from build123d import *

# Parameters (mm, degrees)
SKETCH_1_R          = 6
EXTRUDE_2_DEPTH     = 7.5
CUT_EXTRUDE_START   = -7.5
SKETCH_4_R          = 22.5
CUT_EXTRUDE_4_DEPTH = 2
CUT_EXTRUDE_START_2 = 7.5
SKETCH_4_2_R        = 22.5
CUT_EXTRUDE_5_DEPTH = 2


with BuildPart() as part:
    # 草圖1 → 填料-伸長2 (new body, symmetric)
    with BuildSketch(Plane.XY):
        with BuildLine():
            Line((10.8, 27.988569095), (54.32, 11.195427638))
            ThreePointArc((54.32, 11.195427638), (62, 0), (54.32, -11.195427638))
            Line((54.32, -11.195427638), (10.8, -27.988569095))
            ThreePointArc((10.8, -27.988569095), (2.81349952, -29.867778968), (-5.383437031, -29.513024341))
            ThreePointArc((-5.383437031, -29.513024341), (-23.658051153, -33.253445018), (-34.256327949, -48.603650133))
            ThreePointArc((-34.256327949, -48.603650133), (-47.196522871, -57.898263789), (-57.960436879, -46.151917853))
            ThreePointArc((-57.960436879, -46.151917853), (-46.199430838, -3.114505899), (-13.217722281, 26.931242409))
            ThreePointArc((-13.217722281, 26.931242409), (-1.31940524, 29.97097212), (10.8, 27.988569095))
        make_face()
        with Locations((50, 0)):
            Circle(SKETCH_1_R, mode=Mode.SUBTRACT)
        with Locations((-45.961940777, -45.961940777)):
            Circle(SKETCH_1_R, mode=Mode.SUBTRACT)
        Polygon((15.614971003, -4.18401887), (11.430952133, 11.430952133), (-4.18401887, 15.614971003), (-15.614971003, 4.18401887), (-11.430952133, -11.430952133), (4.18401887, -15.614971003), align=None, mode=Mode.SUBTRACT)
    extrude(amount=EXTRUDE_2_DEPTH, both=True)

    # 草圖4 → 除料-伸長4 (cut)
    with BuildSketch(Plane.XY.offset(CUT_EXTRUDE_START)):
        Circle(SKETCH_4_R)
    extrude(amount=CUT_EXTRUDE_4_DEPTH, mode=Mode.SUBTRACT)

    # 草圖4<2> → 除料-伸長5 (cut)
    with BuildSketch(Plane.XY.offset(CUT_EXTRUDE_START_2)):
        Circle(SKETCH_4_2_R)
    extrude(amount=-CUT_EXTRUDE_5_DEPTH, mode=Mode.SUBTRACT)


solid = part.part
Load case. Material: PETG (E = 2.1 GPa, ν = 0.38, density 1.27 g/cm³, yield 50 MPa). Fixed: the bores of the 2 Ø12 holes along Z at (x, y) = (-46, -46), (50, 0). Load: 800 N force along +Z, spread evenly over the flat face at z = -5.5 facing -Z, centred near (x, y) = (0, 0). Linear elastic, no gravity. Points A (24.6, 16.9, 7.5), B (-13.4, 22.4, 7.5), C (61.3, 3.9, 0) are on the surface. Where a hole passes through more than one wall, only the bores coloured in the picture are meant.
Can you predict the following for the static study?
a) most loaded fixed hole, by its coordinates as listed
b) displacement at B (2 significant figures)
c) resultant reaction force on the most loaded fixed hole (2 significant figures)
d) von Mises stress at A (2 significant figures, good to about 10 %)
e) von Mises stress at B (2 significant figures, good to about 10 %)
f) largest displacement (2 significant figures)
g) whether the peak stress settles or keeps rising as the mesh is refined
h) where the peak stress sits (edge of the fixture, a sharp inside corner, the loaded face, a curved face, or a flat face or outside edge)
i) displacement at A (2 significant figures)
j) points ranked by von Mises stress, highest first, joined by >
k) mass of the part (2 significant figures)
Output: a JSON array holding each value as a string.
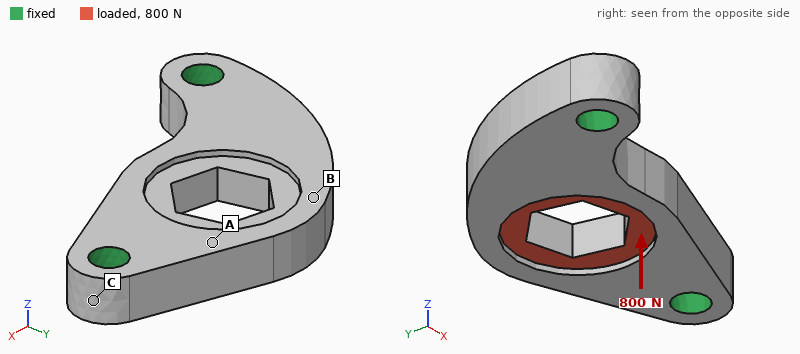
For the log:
["(50, 0)", "0.68 mm", "500 N", "3.5 MPa", "6.5 MPa", "0.73 mm", "keeps rising", "edge of the fixture", "0.26 mm", "B > A > C", "84 g"]
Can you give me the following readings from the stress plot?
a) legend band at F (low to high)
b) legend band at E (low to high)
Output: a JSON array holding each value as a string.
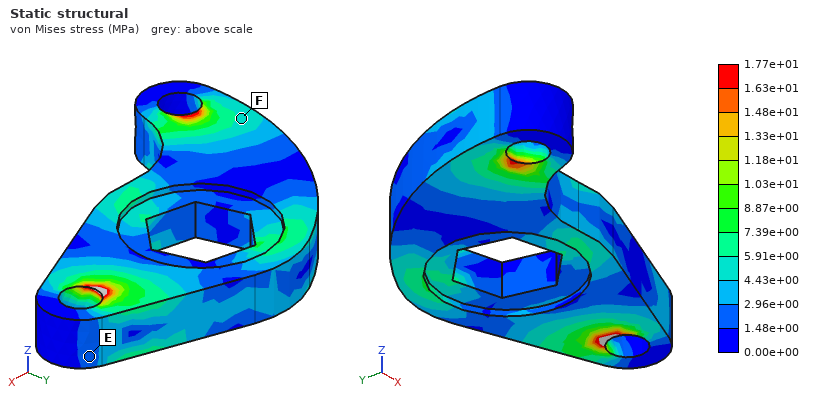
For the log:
["4.43e+00 to 5.91e+00 MPa", "1.48e+00 to 2.96e+00 MPa"]
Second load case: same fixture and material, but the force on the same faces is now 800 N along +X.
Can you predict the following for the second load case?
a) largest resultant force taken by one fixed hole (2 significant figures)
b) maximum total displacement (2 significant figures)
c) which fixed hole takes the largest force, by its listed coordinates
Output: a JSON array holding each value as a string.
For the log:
["610 N", "0.12 mm", "(50, 0)"]
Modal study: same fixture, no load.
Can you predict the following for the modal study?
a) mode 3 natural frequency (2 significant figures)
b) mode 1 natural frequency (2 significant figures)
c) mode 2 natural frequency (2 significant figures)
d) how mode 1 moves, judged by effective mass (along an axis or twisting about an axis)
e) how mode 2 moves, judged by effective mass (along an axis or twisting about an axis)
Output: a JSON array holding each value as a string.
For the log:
["2300 Hz", "920 Hz", "1900 Hz", "along Z", "along Z"]
